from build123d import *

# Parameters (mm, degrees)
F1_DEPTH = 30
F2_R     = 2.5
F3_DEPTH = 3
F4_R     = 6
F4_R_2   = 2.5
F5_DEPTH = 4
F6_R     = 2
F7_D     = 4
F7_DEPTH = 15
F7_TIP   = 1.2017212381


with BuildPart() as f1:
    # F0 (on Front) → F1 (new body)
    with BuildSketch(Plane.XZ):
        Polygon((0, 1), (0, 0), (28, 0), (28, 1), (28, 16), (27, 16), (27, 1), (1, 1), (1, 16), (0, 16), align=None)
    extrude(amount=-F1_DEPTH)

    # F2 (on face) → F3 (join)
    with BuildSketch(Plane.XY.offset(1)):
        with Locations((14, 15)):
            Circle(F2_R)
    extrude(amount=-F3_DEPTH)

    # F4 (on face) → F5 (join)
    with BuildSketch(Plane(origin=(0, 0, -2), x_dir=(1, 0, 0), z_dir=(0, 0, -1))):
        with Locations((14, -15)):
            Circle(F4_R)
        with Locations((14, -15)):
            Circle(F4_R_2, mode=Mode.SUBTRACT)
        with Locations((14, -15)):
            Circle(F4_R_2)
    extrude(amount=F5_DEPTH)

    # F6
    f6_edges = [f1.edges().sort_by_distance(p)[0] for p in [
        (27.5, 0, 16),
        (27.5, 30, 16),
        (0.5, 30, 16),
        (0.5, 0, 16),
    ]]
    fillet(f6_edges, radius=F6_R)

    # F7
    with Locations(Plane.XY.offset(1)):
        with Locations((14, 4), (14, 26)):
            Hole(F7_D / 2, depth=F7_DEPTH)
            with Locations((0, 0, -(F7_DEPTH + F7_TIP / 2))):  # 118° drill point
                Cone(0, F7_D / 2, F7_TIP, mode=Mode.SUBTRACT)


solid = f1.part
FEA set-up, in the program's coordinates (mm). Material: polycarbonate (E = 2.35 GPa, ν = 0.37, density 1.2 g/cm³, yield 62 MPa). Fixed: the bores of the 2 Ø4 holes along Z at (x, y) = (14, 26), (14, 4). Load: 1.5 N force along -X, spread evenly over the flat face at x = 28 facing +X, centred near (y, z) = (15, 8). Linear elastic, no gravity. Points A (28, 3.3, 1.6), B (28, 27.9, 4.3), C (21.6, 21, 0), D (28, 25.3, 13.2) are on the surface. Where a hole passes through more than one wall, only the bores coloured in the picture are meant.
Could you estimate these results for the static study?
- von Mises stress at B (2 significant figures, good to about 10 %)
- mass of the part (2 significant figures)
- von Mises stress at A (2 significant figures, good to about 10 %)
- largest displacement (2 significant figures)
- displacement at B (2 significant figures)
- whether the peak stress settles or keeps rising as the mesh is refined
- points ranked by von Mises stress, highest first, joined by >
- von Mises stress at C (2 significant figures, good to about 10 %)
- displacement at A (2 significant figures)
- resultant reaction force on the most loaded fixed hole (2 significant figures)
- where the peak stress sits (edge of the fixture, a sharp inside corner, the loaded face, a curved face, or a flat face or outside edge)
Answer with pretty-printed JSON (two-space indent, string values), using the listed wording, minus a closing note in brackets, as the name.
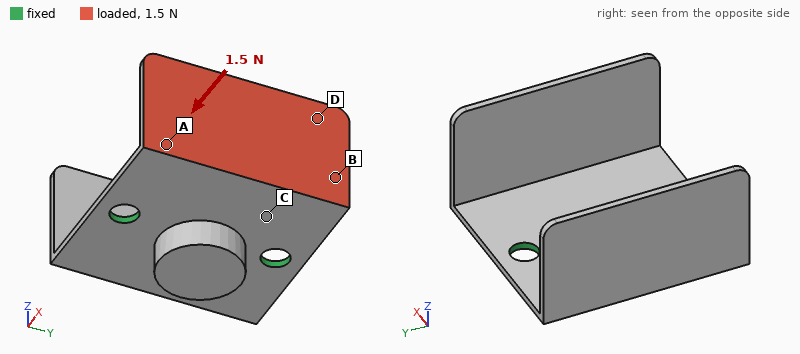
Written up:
{
  "von Mises stress at B": "1.1 MPa",
  "mass of the part": "2.6 g",
  "von Mises stress at A": "1.5 MPa",
  "largest displacement": "0.45 mm",
  "displacement at B": "0.17 mm",
  "whether the peak stress settles or keeps rising as the mesh is refined": "keeps rising",
  "points ranked by von Mises stress, highest first, joined by >": "C > A > B > D",
  "von Mises stress at C": "1.9 MPa",
  "displacement at A": "0.15 mm",
  "resultant reaction force on the most loaded fixed hole": "0.79 N",
  "where the peak stress sits": "edge of the fixture"
}
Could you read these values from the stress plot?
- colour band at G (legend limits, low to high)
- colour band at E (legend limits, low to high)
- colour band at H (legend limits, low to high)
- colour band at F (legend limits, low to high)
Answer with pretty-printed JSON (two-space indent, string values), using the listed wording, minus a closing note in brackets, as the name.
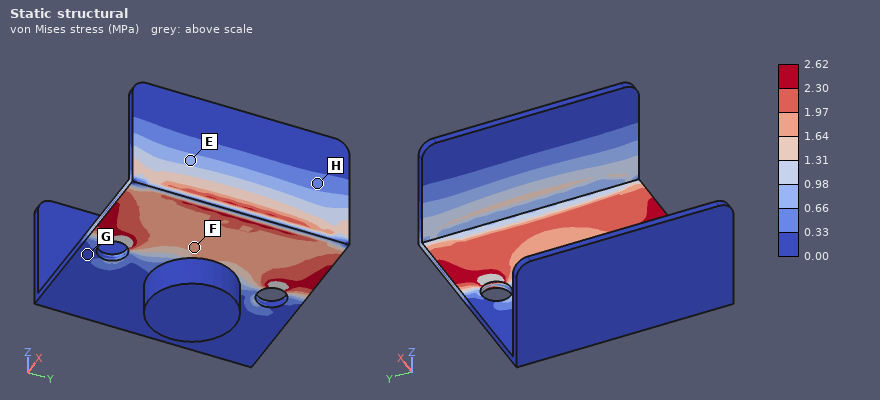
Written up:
{
  "colour band at G": "0.00 to 0.33 MPa",
  "colour band at E": "0.66 to 0.98 MPa",
  "colour band at H": "0.33 to 0.66 MPa",
  "colour band at F": "1.64 to 1.97 MPa"
}
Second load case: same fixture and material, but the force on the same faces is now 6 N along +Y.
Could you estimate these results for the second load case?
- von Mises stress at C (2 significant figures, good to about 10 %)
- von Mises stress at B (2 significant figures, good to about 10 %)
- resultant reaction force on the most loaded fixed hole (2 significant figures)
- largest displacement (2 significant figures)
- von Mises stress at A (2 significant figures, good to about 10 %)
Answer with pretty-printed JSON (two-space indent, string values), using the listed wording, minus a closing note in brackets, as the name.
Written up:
{
  "von Mises stress at C": "2.7 MPa",
  "von Mises stress at B": "2.1 MPa",
  "resultant reaction force on the most loaded fixed hole": "4.9 N",
  "largest displacement": "0.42 mm",
  "von Mises stress at A": "3.0 MPa"
}
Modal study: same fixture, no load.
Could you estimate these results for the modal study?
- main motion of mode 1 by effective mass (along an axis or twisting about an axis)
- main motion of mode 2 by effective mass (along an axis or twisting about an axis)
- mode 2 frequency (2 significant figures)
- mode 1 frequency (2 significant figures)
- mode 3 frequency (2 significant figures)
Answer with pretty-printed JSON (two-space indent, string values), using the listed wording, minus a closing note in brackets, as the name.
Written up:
{
  "main motion of mode 1 by effective mass": "along X",
  "main motion of mode 2 by effective mass": "along Z",
  "mode 2 frequency": "420 Hz",
  "mode 1 frequency": "390 Hz",
  "mode 3 frequency": "740 Hz"
}
